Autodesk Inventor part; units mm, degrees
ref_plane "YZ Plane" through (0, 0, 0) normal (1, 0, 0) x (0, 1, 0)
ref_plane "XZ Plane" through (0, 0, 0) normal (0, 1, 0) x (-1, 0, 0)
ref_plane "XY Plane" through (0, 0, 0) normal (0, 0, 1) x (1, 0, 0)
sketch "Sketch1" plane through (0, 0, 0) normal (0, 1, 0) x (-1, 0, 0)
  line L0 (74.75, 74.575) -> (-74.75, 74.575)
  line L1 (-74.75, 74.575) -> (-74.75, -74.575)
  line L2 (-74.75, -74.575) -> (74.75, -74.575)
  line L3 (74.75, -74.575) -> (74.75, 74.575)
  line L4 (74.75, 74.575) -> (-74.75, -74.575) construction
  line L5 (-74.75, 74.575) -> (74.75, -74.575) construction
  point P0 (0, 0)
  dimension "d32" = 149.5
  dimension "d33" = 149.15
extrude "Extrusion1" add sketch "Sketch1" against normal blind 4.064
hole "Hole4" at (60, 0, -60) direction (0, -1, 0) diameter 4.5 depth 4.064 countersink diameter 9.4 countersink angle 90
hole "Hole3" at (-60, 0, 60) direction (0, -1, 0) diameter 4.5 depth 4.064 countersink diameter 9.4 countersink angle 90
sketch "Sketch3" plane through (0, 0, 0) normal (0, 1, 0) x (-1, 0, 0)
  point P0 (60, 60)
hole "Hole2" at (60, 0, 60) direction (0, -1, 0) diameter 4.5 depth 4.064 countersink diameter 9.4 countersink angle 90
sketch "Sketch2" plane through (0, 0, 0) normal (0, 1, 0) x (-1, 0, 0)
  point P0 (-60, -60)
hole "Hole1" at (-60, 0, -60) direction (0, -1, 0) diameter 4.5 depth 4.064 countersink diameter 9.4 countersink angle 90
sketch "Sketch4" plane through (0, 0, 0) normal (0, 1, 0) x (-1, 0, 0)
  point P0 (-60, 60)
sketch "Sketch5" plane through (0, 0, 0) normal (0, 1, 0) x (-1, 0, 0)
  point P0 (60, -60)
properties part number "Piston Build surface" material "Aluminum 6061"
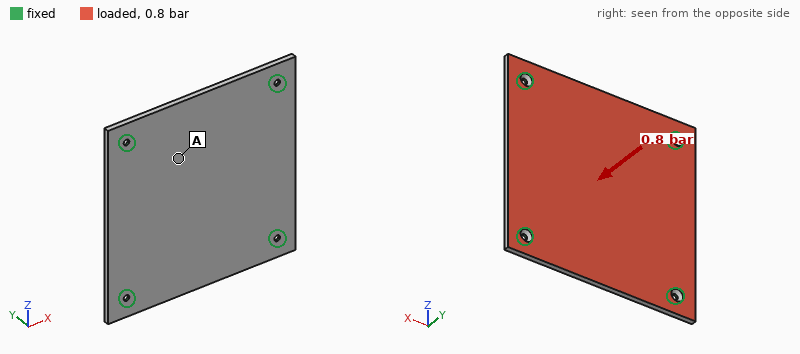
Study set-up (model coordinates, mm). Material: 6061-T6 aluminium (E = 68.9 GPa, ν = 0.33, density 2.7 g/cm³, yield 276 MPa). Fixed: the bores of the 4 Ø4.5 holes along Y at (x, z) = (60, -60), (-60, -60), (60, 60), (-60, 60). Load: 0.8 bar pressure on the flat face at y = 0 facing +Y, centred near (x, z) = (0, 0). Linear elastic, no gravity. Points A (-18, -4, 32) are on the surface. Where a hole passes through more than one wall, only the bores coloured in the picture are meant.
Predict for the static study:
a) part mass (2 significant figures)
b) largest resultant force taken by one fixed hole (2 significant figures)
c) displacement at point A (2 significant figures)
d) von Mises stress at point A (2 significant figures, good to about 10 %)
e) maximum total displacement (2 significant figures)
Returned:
240 g
1.1 kN
0.32 mm
20 MPa
0.40 mm
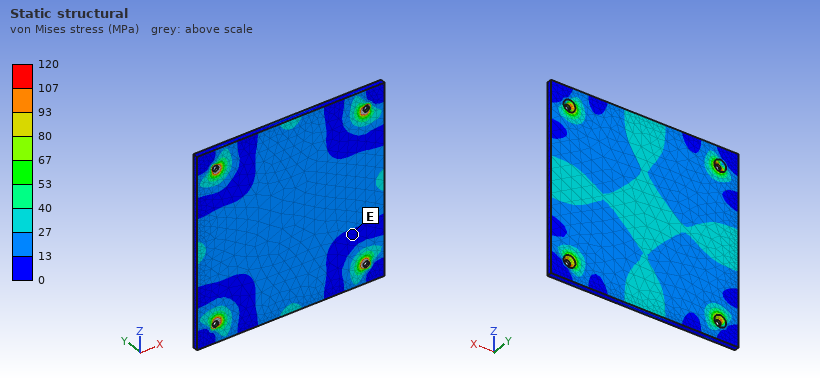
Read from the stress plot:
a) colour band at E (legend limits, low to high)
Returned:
0 to 13 MPa
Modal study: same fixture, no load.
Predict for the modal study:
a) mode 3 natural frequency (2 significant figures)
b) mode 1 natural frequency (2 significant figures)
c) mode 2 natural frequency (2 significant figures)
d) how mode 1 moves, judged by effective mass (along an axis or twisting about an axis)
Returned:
1400 Hz
820 Hz
1400 Hz
along Y
